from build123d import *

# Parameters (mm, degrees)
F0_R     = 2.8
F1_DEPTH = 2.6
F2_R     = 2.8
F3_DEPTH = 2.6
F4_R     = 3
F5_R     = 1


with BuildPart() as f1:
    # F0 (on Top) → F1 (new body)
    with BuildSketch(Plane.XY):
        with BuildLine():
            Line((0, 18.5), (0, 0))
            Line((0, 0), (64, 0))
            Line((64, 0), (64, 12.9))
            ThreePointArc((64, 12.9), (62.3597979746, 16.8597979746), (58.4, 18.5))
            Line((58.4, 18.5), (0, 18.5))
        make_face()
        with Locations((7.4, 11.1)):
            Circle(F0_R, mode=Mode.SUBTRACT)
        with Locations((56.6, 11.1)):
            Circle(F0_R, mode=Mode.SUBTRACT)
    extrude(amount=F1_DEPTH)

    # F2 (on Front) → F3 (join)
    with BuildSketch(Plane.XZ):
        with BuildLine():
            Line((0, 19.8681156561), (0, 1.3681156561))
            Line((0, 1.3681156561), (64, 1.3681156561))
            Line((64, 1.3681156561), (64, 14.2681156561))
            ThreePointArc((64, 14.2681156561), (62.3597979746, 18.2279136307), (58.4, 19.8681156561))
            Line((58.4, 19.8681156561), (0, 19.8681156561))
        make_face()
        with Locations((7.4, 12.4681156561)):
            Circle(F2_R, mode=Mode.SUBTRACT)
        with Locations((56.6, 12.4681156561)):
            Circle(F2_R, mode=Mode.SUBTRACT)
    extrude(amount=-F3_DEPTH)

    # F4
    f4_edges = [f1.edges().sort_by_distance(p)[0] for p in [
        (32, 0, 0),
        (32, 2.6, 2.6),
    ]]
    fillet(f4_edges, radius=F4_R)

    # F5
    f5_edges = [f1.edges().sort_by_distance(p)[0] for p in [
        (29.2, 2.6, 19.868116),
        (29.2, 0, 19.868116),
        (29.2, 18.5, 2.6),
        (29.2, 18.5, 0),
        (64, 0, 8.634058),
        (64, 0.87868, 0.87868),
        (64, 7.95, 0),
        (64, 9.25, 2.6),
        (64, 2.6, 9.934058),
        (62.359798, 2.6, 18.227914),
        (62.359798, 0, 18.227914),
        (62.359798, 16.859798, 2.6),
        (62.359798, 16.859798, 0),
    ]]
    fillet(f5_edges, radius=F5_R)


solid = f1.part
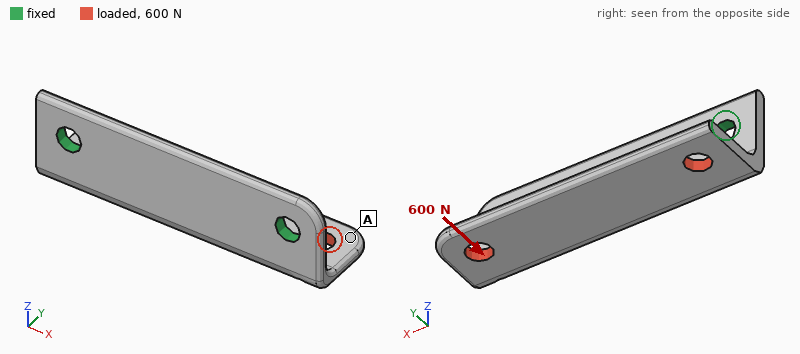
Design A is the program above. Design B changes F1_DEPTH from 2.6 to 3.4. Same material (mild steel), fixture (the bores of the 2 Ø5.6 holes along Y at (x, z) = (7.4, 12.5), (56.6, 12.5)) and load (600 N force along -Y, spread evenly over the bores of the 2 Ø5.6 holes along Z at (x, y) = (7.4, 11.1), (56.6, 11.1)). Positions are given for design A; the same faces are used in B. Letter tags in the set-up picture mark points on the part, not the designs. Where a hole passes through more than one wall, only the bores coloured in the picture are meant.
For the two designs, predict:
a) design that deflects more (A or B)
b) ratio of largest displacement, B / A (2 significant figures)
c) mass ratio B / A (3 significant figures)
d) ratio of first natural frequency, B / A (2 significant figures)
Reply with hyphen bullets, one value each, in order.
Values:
- A
- 0.89
- 1.14
- 0.94
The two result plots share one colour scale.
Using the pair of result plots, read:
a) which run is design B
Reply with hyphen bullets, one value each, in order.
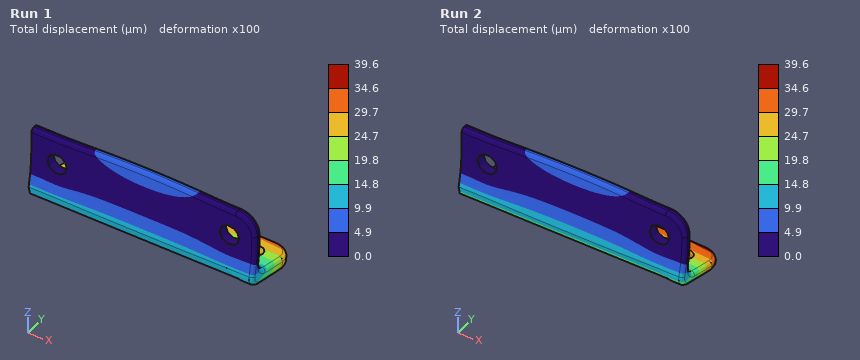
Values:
- Run 1
